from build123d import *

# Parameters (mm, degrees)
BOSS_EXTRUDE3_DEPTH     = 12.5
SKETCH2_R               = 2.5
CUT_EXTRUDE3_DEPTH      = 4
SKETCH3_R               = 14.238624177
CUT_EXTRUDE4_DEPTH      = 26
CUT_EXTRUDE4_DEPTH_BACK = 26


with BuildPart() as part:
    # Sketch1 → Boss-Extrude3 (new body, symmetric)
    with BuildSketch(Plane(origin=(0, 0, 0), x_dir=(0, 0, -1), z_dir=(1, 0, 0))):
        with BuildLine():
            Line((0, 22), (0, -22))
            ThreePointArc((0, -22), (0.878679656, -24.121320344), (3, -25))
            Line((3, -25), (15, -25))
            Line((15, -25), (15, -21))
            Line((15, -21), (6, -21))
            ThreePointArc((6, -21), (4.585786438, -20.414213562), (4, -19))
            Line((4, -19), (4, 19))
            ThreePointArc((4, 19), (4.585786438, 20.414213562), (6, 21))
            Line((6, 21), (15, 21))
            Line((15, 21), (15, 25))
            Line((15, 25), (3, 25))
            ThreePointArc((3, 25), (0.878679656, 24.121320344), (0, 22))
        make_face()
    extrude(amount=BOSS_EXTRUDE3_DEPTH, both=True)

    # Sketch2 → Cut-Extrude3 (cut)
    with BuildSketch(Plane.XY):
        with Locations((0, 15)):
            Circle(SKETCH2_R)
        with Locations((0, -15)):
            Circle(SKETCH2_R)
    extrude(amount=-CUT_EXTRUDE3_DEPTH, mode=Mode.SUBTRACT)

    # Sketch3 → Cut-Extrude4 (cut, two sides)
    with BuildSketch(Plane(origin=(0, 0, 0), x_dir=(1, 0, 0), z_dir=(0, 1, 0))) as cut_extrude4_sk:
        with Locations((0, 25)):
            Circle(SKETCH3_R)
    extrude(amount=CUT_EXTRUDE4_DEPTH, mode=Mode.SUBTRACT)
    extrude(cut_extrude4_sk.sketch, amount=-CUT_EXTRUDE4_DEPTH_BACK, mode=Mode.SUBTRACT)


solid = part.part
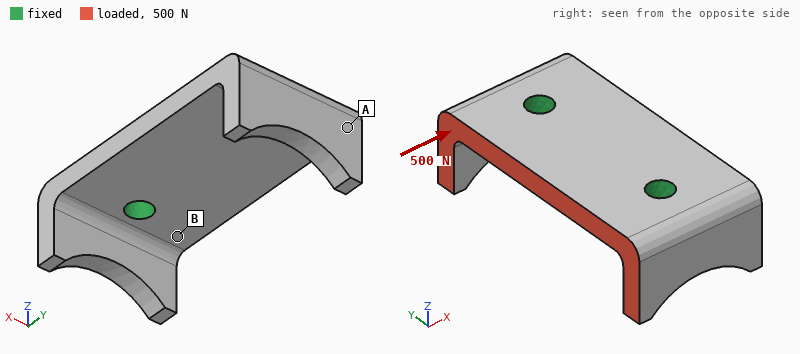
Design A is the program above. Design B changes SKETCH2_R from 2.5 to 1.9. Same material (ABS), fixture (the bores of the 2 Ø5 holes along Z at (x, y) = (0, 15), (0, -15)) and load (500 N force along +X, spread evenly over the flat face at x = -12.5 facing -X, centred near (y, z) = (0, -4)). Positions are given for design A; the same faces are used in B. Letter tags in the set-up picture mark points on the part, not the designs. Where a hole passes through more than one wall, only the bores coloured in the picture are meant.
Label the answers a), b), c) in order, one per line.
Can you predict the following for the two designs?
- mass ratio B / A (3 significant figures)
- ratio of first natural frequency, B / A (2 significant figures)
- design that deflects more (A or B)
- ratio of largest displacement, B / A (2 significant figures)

a) 1.01
b) 0.87
c) B
d) 1.2
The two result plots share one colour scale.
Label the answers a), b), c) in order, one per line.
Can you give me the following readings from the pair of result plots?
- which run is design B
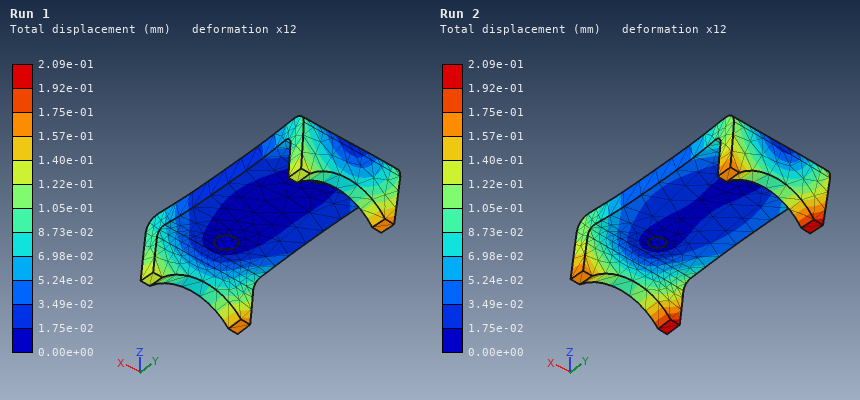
a) Run 2
